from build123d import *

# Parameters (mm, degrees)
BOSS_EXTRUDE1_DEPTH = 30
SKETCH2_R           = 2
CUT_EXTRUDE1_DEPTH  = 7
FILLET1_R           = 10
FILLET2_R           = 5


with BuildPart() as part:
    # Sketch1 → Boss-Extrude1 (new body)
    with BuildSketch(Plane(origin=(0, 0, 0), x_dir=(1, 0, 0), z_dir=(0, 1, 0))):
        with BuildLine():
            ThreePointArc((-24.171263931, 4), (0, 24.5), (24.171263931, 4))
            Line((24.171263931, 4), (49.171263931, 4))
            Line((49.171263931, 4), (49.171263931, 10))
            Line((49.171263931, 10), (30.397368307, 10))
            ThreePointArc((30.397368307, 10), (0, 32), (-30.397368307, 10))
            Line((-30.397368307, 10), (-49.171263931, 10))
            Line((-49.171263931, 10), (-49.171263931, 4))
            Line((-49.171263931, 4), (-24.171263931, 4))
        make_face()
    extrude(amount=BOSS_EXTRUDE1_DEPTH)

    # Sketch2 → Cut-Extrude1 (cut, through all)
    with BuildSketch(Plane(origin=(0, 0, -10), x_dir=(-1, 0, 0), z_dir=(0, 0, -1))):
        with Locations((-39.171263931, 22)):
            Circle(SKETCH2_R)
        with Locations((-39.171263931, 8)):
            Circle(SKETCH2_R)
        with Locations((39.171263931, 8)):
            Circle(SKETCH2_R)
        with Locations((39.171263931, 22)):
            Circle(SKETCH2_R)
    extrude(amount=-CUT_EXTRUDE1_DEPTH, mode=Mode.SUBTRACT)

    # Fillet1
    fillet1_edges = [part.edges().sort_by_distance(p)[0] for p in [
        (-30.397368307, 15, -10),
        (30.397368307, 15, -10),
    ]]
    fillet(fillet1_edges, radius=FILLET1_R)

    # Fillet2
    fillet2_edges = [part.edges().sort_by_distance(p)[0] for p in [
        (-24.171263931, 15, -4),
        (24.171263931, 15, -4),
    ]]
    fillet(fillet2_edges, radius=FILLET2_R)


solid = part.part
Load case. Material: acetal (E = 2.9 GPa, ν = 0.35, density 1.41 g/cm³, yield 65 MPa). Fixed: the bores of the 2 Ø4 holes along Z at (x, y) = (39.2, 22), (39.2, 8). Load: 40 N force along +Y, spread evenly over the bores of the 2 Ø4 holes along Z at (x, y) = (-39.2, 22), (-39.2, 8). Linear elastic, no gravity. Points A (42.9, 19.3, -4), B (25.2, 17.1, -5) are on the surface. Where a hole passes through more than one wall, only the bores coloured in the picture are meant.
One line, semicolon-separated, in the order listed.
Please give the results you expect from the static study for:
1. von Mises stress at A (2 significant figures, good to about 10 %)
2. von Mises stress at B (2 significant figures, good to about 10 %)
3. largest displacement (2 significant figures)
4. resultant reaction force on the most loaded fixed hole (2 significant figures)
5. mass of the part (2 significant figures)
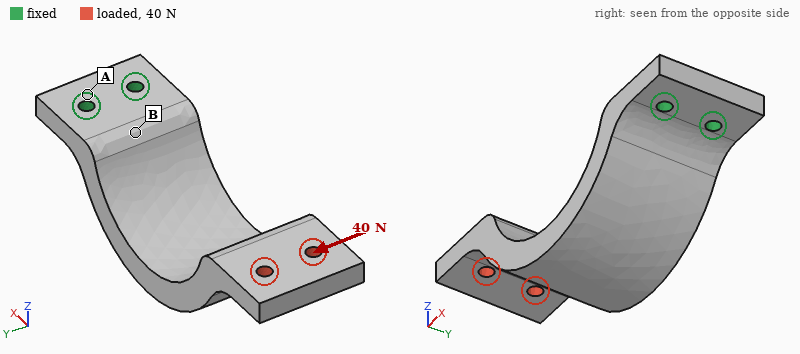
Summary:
1.1 MPa; 4.2 MPa; 1.0 mm; 190 N; 35 g
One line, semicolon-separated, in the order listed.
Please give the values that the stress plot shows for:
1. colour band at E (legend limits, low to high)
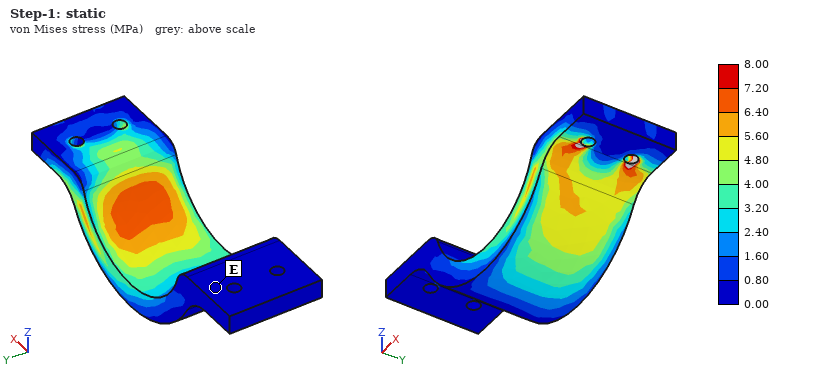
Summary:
0.00 to 0.80 MPa
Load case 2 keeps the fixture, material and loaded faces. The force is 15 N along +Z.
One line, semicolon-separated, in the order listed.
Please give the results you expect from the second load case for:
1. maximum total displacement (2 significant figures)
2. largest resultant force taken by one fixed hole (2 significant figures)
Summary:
1.3 mm; 9.2 N
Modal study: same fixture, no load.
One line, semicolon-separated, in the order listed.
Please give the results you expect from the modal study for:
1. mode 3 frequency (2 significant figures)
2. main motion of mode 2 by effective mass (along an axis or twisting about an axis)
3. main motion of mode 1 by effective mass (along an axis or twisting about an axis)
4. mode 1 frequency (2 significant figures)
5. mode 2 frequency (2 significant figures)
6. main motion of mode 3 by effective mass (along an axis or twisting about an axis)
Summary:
680 Hz; along Y; along Z; 180 Hz; 360 Hz; along X
